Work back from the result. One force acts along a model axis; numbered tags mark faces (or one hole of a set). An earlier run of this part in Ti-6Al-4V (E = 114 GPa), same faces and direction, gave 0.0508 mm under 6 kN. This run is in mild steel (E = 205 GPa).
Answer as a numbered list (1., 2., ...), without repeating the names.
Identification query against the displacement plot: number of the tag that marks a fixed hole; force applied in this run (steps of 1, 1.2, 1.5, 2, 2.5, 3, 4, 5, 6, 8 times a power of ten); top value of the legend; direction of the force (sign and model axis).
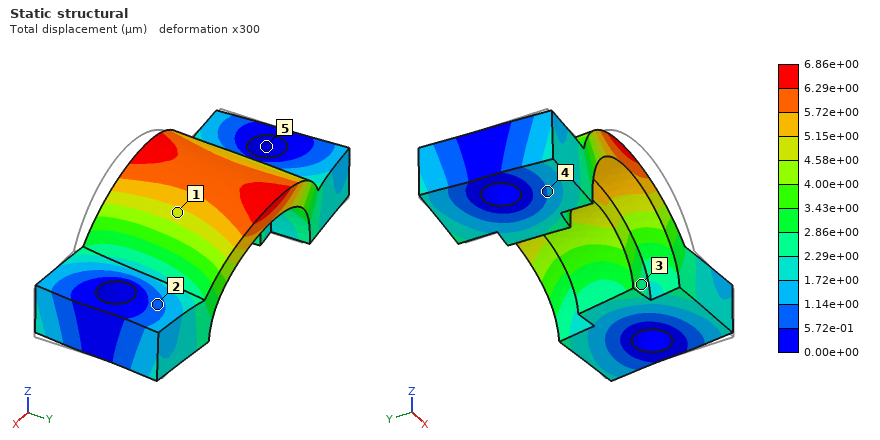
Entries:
1. 5
2. 1.5 kN
3. 6.86e+00 µm
4. +Y
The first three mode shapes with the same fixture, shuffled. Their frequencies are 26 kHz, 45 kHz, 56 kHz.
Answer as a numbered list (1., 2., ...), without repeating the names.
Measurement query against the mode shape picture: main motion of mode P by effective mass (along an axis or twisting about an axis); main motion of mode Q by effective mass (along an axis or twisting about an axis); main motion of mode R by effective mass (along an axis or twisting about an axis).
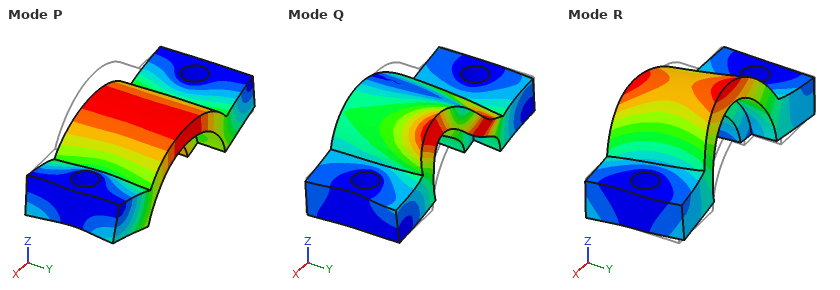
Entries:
1. along Z
2. along X
3. along Y
